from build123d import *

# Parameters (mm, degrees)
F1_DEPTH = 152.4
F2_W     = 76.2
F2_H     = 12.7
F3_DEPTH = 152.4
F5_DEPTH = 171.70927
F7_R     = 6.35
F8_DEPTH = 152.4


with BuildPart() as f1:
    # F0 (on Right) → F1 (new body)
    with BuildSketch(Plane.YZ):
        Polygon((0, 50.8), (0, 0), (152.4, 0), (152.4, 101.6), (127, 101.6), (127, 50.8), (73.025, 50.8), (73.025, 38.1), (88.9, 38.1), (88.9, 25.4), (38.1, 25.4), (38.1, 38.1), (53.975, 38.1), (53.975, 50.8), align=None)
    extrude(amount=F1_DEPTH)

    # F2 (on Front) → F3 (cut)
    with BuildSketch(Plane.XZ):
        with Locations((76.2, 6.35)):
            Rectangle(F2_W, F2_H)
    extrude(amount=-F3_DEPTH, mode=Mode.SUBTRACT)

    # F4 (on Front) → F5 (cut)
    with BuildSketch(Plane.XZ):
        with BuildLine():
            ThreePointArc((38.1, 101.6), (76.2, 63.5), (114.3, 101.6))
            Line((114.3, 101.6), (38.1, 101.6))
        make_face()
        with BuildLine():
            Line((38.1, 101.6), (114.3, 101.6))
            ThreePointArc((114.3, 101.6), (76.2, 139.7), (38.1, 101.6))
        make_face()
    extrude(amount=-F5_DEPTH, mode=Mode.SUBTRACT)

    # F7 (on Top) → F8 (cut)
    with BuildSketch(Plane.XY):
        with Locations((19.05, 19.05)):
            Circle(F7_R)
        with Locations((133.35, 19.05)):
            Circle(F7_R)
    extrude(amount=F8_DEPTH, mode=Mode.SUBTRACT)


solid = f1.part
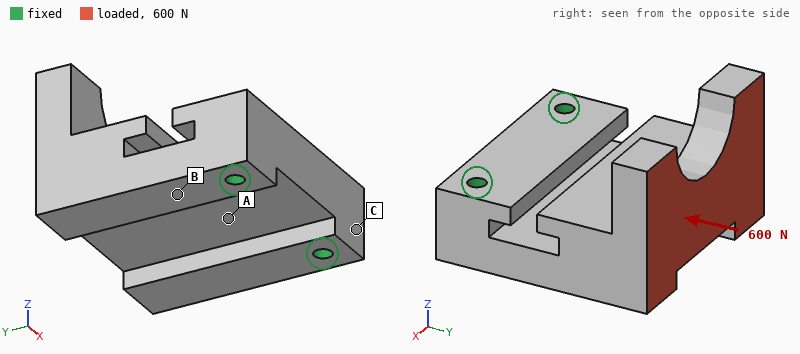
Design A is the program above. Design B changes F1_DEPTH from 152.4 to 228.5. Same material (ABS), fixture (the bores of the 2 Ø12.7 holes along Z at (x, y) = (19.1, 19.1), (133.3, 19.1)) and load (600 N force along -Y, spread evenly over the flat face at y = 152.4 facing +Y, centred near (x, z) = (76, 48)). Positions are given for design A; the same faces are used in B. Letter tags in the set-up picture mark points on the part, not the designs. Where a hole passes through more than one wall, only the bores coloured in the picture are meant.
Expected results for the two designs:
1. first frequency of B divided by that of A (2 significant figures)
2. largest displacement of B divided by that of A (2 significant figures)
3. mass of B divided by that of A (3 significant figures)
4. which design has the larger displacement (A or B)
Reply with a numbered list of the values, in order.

1. 0.96
2. 0.67
3. 1.61
4. A
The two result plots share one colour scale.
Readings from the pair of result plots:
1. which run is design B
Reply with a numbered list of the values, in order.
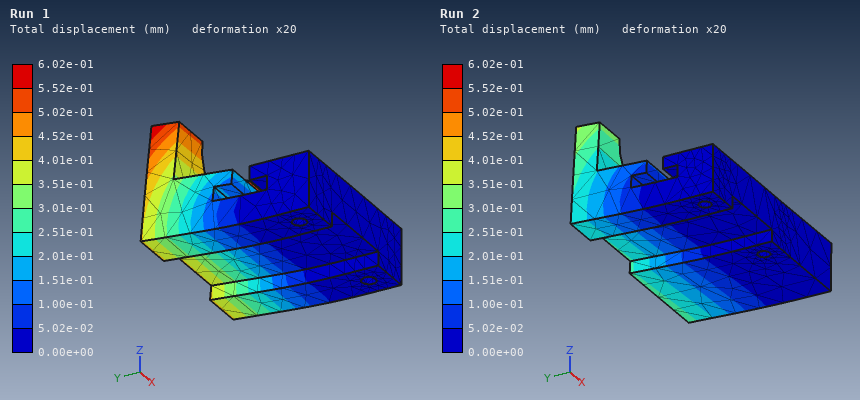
1. Run 2
